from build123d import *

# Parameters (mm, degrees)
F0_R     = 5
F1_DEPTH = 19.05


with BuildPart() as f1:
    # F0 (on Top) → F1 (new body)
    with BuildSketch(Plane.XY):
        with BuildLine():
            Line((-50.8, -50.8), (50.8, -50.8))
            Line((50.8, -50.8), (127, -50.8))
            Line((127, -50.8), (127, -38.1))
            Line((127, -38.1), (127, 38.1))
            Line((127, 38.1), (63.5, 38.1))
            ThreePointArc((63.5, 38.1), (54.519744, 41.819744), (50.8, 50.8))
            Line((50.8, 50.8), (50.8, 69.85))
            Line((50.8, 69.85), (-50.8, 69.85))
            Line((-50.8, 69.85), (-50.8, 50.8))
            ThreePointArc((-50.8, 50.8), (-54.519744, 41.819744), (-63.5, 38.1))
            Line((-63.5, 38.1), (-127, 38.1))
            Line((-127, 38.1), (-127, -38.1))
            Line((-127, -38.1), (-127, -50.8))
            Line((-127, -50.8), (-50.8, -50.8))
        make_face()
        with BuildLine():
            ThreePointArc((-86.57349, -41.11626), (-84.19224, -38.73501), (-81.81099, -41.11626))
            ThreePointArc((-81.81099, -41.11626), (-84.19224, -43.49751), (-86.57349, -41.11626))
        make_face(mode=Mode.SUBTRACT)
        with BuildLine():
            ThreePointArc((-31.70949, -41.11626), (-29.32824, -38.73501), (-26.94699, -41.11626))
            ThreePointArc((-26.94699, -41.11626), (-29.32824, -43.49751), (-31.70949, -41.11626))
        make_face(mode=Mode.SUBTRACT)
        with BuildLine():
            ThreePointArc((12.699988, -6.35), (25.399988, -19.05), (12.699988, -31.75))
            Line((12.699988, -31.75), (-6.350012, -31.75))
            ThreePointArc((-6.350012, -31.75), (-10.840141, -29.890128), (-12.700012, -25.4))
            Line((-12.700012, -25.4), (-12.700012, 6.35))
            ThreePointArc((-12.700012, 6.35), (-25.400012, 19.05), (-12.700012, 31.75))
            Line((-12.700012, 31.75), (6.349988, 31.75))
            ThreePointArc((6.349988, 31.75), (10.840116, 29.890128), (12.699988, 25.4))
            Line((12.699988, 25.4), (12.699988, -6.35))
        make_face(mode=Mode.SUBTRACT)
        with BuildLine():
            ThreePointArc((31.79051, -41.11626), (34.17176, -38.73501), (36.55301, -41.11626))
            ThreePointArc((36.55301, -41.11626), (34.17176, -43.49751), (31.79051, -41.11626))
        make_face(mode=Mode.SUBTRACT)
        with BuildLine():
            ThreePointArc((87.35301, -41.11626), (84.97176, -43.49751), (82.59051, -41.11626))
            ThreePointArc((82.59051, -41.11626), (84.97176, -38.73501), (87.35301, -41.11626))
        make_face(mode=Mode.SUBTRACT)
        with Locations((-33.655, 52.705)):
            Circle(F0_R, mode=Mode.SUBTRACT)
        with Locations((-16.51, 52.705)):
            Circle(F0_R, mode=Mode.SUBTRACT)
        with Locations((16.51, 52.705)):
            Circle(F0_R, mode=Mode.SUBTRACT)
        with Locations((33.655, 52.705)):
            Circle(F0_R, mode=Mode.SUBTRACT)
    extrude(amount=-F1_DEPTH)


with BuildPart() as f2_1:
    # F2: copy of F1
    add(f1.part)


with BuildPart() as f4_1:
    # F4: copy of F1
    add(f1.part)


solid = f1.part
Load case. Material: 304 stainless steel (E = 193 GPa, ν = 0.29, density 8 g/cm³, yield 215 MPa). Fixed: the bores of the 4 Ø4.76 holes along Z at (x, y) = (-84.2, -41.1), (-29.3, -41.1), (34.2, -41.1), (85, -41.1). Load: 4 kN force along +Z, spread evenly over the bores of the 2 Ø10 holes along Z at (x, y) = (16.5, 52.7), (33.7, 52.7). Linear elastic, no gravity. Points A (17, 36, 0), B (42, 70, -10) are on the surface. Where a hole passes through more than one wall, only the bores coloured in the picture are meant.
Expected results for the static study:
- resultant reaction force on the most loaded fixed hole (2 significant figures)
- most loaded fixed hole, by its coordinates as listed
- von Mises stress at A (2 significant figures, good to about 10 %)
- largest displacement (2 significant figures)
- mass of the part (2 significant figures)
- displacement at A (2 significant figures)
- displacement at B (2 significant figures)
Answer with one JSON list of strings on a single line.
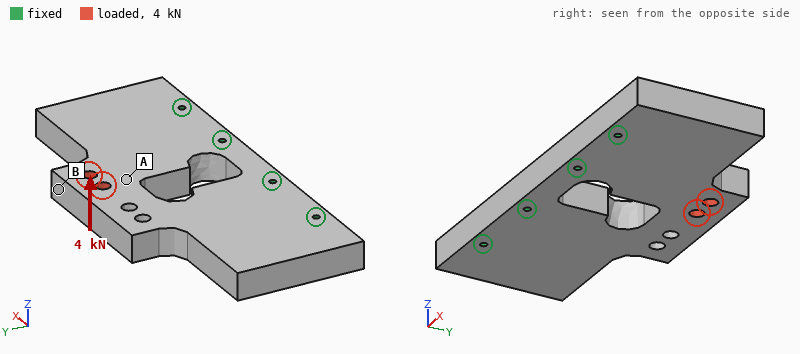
["1.7 kN", "(34.2, -41.1)", "26 MPa", "0.13 mm", "3.6 kg", "0.076 mm", "0.13 mm"]
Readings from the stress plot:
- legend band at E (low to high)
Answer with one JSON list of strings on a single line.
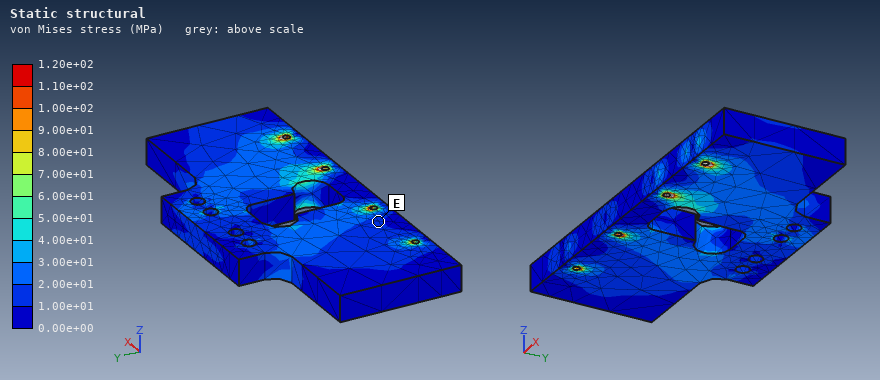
["1.00e+01 to 2.00e+01 MPa"]
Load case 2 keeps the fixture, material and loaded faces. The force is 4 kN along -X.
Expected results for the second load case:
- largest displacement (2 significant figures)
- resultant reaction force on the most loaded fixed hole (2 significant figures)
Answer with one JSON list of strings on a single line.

["4.9 µm", "2.8 kN"]
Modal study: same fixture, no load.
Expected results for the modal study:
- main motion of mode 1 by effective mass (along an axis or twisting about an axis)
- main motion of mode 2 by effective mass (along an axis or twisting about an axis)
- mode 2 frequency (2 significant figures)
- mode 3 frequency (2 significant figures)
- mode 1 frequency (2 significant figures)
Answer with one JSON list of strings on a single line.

["along Z", "twisting about Y", "1900 Hz", "2700 Hz", "1200 Hz"]
